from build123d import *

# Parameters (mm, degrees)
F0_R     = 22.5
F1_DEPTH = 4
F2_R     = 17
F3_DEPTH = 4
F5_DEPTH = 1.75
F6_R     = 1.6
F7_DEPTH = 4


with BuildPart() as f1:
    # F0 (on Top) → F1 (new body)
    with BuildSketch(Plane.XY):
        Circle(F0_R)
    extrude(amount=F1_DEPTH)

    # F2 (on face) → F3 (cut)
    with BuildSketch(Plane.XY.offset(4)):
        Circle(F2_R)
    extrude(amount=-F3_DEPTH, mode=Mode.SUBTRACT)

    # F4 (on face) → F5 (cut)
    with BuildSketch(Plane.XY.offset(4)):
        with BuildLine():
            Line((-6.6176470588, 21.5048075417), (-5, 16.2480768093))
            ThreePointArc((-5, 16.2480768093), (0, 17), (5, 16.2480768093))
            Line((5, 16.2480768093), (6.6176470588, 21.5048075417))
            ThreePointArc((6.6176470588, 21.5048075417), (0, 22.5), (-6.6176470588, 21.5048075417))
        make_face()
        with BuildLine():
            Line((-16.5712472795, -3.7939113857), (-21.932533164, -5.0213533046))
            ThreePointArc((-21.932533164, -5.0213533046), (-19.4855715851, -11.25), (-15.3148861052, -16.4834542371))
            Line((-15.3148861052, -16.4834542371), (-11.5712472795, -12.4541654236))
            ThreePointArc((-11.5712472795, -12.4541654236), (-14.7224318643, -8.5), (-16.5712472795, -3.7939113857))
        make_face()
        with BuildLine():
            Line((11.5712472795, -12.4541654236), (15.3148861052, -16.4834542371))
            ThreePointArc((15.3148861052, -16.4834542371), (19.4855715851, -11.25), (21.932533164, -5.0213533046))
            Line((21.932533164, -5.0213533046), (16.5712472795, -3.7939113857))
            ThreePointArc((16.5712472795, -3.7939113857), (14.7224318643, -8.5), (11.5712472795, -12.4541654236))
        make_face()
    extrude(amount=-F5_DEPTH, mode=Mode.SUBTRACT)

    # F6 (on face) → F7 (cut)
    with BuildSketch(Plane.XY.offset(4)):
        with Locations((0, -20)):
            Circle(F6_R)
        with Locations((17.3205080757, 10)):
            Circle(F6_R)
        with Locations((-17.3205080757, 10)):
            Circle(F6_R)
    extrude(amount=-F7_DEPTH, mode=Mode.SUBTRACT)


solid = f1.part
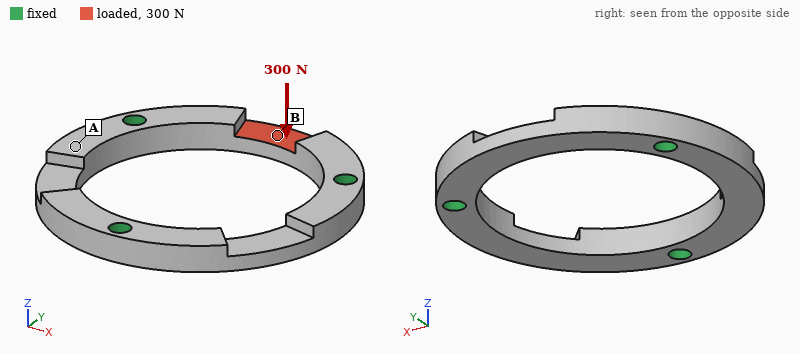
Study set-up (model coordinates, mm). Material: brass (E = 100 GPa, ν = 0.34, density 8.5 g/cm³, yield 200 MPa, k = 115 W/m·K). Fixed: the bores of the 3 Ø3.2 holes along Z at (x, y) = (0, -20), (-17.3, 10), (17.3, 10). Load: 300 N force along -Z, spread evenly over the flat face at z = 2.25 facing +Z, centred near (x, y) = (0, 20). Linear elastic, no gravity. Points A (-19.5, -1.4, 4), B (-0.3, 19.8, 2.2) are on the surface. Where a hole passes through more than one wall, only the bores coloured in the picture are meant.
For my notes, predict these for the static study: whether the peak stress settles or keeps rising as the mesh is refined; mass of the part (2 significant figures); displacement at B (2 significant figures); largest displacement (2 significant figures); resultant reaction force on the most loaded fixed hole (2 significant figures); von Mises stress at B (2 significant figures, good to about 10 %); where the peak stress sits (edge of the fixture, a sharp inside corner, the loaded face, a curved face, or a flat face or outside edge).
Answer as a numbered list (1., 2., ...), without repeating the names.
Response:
1. keeps rising
2. 19 g
3. 62 µm
4. 73 µm
5. 160 N
6. 94 MPa
7. edge of the fixture
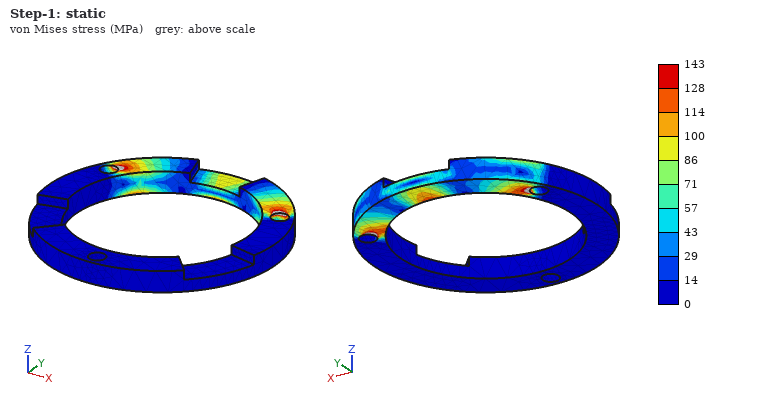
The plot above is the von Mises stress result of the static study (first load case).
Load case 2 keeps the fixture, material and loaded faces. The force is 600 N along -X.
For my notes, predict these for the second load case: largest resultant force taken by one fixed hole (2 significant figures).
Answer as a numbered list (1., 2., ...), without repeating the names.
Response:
1. 320 N
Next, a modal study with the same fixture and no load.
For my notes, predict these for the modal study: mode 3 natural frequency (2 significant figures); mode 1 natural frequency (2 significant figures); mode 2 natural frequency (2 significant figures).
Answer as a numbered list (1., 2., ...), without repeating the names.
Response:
1. 7900 Hz
2. 7800 Hz
3. 7800 Hz
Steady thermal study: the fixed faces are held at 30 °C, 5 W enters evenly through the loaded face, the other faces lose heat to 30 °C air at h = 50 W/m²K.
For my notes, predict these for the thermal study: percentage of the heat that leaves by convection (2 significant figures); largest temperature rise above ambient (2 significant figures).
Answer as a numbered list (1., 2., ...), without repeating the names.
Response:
1. 5.6 %
2. 19 K
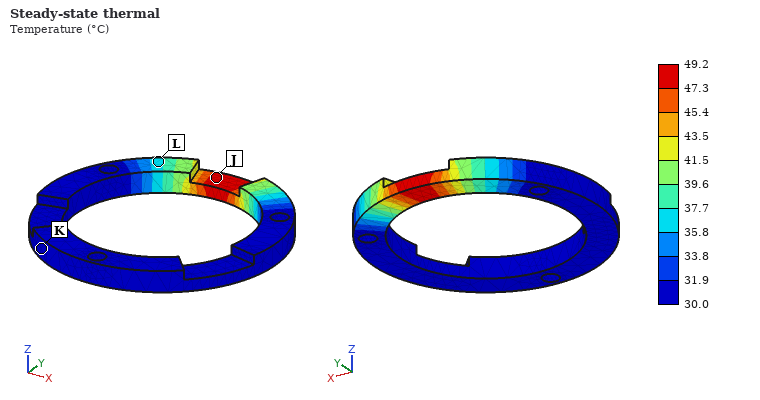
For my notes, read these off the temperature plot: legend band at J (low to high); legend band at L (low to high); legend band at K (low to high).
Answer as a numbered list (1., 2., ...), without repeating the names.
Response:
1. 47.3 to 49.2 °C
2. 35.8 to 37.7 °C
3. 30.0 to 31.9 °C
